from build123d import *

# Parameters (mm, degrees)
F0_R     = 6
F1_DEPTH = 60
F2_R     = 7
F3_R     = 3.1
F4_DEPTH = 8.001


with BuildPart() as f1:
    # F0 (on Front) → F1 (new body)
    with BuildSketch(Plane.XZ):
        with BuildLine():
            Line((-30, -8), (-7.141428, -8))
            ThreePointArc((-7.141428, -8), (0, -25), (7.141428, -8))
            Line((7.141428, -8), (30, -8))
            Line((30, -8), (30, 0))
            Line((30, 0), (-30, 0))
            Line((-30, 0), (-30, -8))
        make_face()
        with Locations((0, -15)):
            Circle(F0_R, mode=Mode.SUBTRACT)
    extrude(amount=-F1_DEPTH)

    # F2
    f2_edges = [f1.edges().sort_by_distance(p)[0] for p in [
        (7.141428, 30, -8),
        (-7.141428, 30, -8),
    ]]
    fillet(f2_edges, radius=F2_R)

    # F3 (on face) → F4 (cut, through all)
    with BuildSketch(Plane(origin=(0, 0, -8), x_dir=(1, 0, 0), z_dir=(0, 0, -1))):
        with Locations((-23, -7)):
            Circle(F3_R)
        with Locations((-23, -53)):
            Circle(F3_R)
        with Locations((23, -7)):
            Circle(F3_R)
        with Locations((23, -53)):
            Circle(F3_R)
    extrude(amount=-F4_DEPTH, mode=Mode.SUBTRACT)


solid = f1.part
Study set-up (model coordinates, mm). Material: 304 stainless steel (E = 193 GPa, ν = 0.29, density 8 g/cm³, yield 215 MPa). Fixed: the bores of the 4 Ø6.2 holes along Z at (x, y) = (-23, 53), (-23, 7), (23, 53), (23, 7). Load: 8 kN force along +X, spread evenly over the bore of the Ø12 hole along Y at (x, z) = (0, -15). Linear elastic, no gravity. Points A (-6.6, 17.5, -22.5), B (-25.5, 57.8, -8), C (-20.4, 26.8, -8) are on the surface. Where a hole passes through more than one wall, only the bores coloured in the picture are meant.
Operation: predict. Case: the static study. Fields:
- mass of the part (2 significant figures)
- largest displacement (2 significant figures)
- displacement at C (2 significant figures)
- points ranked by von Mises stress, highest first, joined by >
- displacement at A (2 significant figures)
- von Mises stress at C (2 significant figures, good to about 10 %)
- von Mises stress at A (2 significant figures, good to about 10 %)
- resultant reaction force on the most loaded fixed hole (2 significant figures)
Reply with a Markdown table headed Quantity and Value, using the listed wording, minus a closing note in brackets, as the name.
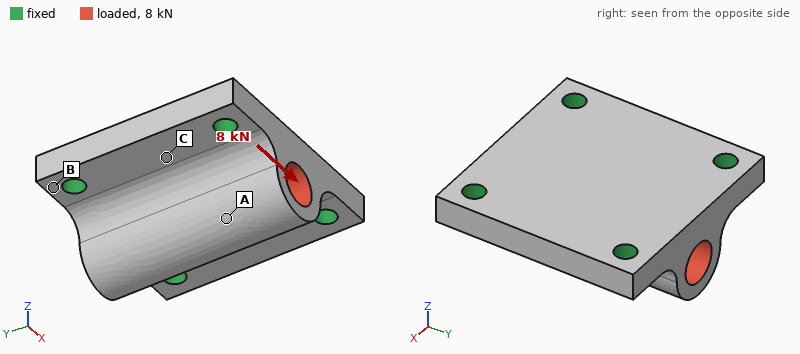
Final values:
| Quantity | Value |
|---|---|
| mass of the part | 320 g |
| largest displacement | 6.7 µm |
| displacement at C | 2.1 µm |
| points ranked by von Mises stress, highest first, joined by > | A > C > B |
| displacement at A | 6.5 µm |
| von Mises stress at C | 8.4 MPa |
| von Mises stress at A | 16 MPa |
| resultant reaction force on the most loaded fixed hole | 2.4 kN |
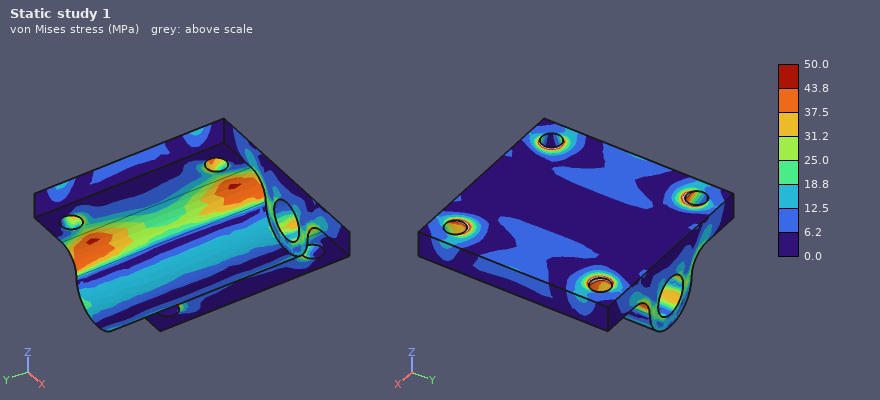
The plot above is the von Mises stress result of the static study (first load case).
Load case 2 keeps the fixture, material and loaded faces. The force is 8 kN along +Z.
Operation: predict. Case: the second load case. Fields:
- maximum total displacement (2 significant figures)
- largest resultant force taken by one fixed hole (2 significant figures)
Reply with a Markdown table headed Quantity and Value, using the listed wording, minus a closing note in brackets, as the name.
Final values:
| Quantity | Value |
|---|---|
| maximum total displacement | 7.2 µm |
| largest resultant force taken by one fixed hole | 2.1 kN |
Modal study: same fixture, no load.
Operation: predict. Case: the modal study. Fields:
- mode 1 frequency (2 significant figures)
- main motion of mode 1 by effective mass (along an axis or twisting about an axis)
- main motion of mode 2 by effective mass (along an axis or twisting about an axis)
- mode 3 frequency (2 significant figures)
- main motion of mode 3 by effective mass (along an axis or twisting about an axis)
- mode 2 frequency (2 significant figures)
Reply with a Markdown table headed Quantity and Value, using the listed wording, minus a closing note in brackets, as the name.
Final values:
| Quantity | Value |
|---|---|
| mode 1 frequency | 12 kHz |
| main motion of mode 1 by effective mass | along Z |
| main motion of mode 2 by effective mass | along Y |
| mode 3 frequency | 17 kHz |
| main motion of mode 3 by effective mass | along X |
| mode 2 frequency | 15 kHz |
